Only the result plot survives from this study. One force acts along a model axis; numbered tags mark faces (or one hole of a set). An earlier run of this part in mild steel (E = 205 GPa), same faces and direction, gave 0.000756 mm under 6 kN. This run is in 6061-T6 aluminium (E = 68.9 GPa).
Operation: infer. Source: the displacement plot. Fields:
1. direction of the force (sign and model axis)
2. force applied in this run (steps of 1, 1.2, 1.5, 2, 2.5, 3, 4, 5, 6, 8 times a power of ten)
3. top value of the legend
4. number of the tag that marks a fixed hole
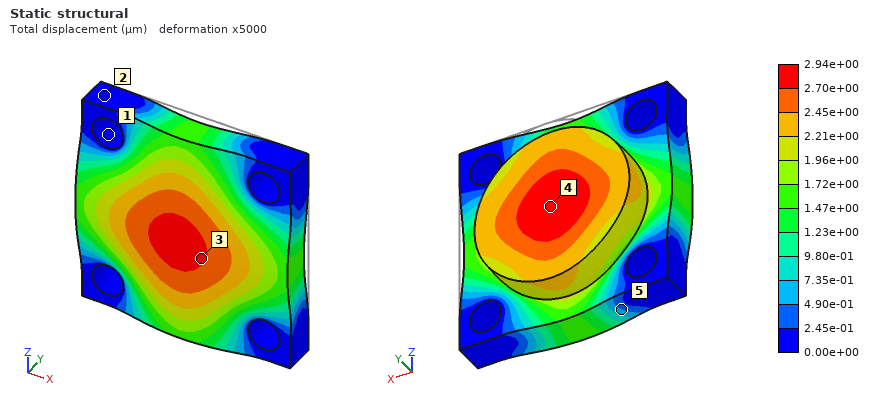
-Y
8 kN
2.94e+00 µm
1
